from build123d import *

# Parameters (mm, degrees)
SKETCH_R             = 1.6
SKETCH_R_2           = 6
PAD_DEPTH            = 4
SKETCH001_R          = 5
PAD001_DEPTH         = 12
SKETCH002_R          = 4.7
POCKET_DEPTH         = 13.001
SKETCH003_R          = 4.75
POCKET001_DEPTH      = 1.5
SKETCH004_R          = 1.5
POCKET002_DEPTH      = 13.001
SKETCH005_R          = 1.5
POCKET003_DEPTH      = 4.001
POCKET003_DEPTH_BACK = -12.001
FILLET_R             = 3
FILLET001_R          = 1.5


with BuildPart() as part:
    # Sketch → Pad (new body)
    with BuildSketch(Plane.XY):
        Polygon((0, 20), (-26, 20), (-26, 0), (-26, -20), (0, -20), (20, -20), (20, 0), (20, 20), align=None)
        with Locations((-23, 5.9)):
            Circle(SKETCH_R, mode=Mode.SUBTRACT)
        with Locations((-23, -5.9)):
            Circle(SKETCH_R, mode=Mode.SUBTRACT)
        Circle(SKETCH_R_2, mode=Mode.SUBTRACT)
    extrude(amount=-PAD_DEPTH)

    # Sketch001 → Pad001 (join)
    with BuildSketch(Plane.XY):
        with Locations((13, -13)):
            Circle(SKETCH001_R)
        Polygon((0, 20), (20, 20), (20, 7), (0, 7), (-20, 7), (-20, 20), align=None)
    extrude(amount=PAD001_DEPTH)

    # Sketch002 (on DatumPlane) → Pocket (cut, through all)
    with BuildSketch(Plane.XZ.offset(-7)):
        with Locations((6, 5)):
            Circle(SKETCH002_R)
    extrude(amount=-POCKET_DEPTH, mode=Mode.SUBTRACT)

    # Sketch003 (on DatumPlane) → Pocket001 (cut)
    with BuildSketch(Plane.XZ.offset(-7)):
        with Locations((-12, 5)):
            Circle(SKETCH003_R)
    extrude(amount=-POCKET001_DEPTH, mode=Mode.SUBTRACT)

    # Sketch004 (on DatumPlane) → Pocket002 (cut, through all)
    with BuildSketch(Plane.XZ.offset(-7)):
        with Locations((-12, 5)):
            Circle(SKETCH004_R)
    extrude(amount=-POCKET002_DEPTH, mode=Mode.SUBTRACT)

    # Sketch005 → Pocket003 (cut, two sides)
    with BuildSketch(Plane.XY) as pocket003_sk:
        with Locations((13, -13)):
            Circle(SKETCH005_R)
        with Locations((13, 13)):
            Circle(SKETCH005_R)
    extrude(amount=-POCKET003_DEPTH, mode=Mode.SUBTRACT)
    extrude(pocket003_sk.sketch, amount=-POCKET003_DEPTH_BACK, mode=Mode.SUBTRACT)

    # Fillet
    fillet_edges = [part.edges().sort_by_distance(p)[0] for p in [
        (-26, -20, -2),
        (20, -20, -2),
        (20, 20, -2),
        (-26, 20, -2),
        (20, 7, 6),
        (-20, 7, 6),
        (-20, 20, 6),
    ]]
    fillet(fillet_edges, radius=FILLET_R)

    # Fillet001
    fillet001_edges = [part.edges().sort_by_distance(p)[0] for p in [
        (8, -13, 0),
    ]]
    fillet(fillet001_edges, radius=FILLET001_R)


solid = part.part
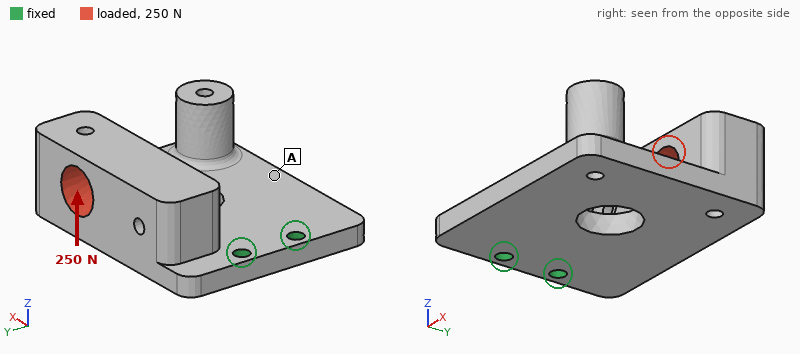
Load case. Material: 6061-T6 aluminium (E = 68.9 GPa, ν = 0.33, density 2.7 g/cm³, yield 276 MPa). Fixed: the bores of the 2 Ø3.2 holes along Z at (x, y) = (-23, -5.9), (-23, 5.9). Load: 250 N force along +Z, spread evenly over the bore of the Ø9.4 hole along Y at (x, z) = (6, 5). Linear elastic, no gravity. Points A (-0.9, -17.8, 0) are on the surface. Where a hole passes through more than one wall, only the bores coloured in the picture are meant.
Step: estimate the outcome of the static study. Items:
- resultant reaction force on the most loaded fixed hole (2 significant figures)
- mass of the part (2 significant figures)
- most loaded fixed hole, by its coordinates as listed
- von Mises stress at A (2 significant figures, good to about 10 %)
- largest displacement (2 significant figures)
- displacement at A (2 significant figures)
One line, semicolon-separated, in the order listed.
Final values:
280 N; 34 g; (-23, 5.9); 18 MPa; 0.27 mm; 0.049 mm
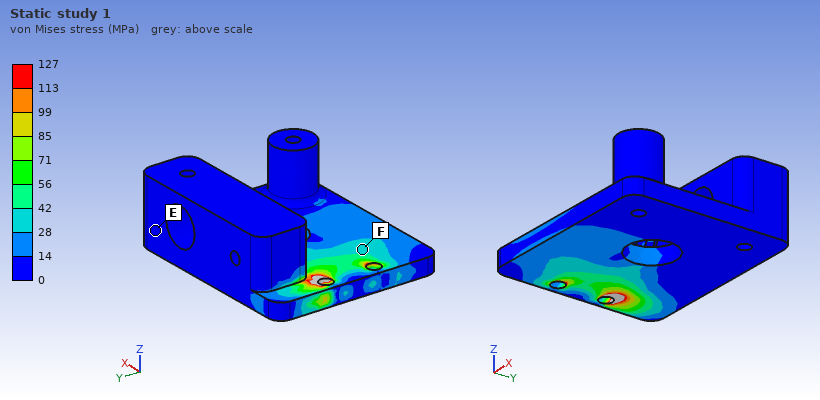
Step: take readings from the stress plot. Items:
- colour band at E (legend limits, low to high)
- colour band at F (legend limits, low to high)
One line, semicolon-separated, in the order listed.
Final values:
0 to 14 MPa; 28 to 42 MPa
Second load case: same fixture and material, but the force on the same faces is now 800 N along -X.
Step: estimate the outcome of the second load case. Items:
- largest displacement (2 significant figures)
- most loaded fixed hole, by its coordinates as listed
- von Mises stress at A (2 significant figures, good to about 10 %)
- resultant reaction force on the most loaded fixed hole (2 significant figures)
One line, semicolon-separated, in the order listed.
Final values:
0.21 mm; (-23, 5.9); 11 MPa; 1.1 kN
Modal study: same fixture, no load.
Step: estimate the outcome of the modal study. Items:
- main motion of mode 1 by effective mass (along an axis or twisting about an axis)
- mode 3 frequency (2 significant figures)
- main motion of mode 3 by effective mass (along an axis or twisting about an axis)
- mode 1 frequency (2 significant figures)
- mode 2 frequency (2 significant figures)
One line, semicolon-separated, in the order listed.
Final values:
along Z; 4300 Hz; along Y; 1300 Hz; 2700 Hz
